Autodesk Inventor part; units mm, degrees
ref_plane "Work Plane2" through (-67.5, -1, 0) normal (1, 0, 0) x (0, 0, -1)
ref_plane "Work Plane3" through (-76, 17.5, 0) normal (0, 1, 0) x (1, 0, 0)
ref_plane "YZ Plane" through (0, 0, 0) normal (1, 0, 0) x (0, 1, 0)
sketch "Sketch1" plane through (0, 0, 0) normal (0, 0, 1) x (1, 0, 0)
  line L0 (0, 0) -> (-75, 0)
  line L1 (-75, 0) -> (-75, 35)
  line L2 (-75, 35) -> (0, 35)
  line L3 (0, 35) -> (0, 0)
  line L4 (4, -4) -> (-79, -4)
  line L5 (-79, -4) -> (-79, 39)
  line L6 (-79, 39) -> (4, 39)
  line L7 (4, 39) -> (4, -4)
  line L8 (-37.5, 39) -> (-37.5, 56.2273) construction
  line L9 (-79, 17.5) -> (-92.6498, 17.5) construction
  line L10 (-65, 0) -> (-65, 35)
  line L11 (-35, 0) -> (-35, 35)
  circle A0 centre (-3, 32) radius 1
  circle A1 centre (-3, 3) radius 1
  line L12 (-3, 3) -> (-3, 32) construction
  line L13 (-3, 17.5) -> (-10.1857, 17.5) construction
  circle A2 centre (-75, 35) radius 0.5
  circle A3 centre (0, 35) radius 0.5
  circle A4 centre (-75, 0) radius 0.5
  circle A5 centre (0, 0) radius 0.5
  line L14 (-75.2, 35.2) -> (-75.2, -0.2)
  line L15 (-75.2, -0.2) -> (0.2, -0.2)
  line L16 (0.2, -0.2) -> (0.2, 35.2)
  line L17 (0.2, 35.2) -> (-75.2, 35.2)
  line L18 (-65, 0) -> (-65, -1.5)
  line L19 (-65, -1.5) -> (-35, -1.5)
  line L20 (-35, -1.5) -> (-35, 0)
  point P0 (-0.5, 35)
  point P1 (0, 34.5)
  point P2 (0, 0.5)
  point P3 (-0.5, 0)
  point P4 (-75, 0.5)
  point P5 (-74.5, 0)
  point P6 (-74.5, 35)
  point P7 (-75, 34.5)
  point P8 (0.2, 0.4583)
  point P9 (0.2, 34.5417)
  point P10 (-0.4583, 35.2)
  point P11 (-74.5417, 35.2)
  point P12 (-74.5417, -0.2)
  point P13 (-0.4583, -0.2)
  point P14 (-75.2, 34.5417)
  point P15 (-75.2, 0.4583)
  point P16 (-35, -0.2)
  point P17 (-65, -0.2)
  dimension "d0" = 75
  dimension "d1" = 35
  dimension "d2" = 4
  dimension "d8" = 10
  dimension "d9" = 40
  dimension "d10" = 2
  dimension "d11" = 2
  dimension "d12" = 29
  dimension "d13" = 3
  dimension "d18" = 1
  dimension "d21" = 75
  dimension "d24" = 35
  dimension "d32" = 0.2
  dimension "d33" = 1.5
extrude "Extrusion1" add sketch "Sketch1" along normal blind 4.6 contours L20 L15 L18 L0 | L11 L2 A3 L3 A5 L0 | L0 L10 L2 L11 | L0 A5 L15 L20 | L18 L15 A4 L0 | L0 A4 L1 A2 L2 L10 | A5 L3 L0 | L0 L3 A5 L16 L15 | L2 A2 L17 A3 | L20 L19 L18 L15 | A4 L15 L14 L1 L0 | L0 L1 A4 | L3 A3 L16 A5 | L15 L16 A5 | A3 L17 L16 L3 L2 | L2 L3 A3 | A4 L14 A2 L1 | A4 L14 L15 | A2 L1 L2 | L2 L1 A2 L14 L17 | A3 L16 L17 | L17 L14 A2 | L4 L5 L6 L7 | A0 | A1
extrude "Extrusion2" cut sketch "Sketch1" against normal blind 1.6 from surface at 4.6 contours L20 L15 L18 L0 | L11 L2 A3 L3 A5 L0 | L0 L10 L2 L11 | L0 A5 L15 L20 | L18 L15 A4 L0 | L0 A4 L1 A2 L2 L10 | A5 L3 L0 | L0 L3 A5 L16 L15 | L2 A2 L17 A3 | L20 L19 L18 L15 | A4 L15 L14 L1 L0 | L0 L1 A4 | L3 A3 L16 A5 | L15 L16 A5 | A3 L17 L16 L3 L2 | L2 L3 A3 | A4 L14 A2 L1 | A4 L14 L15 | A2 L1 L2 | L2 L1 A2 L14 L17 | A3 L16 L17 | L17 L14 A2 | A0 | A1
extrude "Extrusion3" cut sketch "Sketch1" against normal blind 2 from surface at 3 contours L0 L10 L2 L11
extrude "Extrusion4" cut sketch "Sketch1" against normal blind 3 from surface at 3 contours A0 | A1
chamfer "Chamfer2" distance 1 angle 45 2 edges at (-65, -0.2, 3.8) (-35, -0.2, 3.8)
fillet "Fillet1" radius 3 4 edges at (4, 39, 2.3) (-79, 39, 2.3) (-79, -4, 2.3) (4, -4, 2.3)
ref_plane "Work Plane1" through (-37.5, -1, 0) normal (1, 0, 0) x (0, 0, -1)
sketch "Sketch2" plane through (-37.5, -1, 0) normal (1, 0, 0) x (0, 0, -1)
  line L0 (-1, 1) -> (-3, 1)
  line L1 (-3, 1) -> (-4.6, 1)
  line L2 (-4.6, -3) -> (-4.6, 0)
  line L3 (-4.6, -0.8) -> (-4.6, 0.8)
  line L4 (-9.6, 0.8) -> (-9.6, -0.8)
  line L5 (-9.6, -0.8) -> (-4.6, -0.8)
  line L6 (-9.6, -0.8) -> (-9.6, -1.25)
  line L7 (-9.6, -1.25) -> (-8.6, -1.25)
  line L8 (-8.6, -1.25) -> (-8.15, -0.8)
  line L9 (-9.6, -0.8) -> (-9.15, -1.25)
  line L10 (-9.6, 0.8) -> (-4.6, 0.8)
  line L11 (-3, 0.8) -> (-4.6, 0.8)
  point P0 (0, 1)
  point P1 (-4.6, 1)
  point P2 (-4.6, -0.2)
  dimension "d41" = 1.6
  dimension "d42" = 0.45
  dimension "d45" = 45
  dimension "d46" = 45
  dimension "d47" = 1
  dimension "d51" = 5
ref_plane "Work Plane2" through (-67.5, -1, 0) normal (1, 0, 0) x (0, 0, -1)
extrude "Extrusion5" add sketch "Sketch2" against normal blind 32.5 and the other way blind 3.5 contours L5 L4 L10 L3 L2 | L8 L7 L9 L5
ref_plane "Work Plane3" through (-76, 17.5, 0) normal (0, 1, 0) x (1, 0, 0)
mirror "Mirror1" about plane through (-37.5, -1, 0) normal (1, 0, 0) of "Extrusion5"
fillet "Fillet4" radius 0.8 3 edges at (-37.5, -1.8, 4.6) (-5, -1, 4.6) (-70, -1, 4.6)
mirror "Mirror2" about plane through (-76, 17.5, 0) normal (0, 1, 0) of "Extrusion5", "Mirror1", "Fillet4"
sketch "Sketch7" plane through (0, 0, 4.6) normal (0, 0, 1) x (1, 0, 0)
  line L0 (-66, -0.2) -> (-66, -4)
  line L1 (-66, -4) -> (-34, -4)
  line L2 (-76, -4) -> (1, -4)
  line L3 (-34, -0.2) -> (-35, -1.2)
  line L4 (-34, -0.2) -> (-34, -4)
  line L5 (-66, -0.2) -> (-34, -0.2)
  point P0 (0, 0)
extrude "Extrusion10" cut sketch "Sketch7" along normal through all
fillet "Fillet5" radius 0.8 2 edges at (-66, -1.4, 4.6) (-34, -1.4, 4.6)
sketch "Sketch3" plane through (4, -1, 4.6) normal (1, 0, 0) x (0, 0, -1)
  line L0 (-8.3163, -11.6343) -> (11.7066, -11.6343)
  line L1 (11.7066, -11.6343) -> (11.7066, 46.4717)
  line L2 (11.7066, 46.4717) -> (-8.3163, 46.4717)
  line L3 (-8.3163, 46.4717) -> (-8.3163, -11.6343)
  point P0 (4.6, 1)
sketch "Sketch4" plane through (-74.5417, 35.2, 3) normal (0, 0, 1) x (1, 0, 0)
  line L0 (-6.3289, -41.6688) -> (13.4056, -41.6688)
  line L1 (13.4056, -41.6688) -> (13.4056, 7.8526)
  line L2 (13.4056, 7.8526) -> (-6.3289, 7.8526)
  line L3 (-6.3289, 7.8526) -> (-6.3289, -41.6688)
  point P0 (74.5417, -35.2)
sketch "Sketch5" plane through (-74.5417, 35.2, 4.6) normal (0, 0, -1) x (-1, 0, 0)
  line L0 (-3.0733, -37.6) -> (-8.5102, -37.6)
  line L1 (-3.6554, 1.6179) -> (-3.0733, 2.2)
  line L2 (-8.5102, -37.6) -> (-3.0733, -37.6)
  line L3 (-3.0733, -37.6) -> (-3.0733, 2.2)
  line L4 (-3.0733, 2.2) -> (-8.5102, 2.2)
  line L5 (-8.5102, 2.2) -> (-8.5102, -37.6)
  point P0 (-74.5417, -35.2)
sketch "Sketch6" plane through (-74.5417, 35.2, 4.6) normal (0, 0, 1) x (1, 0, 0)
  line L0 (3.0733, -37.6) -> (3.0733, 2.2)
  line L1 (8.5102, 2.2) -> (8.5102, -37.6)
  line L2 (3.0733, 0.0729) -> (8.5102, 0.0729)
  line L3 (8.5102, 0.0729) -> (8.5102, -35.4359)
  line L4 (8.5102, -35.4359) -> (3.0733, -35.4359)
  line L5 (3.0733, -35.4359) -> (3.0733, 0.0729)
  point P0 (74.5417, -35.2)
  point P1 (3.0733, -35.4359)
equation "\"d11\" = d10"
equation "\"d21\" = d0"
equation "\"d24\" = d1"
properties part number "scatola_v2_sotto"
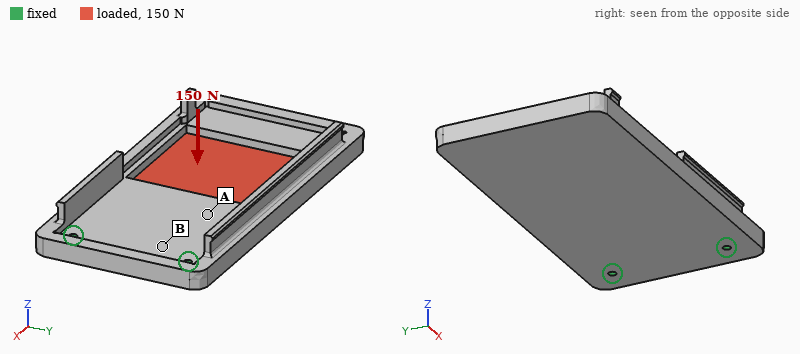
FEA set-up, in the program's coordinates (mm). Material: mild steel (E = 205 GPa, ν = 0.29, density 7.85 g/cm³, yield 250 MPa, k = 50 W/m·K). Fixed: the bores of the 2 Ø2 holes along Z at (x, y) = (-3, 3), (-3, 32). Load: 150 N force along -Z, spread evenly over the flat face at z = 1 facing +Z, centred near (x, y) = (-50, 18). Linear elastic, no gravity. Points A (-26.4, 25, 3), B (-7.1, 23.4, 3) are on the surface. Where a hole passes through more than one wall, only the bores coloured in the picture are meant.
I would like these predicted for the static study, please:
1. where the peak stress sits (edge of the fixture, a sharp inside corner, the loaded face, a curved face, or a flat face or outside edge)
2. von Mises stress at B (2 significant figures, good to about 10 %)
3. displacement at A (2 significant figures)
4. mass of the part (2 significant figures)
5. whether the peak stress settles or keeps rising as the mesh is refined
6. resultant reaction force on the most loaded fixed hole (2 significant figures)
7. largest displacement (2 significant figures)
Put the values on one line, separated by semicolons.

edge of the fixture; 39 MPa; 0.058 mm; 85 g; keeps rising; 82 N; 0.26 mm
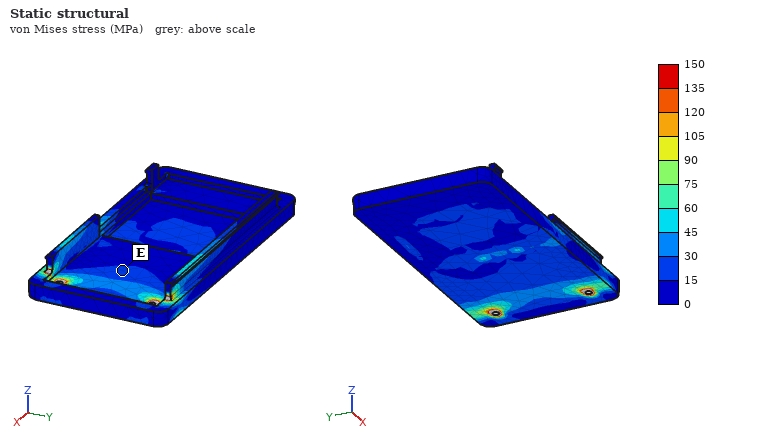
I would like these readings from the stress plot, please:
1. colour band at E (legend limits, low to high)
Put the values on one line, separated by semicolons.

15 to 30 MPa
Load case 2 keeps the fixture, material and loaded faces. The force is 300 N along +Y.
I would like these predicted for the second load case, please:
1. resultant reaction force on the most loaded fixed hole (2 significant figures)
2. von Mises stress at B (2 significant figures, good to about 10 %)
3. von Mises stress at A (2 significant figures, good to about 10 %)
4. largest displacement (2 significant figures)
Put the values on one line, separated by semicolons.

500 N; 5.4 MPa; 7.2 MPa; 13 µm
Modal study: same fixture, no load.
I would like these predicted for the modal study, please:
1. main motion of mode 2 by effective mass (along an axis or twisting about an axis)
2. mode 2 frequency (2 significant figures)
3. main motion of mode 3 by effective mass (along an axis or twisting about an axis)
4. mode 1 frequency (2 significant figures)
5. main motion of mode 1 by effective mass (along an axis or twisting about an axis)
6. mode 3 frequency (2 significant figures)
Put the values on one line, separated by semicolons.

twisting about X; 1400 Hz; along Z; 610 Hz; along Z; 3400 Hz
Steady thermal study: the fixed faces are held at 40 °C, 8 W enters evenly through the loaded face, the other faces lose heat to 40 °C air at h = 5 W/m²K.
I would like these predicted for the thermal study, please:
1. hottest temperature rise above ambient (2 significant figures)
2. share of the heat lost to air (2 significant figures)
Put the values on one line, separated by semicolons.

63 K; 19 %
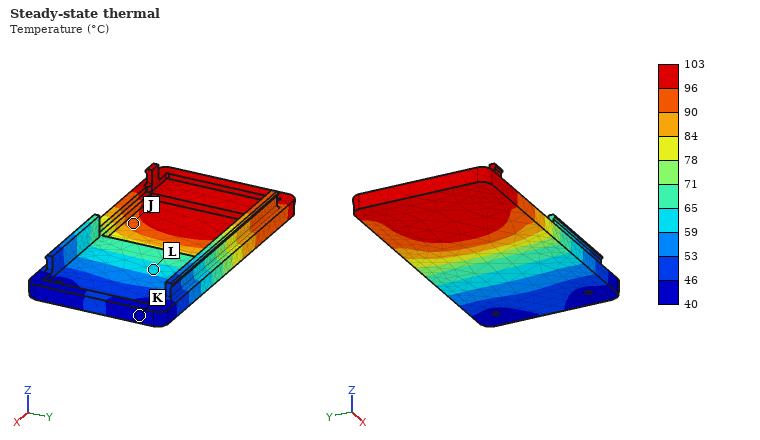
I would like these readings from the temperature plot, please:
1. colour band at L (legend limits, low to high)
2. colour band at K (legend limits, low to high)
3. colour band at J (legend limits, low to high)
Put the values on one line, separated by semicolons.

59 to 65 °C; 40 to 46 °C; 90 to 96 °C
